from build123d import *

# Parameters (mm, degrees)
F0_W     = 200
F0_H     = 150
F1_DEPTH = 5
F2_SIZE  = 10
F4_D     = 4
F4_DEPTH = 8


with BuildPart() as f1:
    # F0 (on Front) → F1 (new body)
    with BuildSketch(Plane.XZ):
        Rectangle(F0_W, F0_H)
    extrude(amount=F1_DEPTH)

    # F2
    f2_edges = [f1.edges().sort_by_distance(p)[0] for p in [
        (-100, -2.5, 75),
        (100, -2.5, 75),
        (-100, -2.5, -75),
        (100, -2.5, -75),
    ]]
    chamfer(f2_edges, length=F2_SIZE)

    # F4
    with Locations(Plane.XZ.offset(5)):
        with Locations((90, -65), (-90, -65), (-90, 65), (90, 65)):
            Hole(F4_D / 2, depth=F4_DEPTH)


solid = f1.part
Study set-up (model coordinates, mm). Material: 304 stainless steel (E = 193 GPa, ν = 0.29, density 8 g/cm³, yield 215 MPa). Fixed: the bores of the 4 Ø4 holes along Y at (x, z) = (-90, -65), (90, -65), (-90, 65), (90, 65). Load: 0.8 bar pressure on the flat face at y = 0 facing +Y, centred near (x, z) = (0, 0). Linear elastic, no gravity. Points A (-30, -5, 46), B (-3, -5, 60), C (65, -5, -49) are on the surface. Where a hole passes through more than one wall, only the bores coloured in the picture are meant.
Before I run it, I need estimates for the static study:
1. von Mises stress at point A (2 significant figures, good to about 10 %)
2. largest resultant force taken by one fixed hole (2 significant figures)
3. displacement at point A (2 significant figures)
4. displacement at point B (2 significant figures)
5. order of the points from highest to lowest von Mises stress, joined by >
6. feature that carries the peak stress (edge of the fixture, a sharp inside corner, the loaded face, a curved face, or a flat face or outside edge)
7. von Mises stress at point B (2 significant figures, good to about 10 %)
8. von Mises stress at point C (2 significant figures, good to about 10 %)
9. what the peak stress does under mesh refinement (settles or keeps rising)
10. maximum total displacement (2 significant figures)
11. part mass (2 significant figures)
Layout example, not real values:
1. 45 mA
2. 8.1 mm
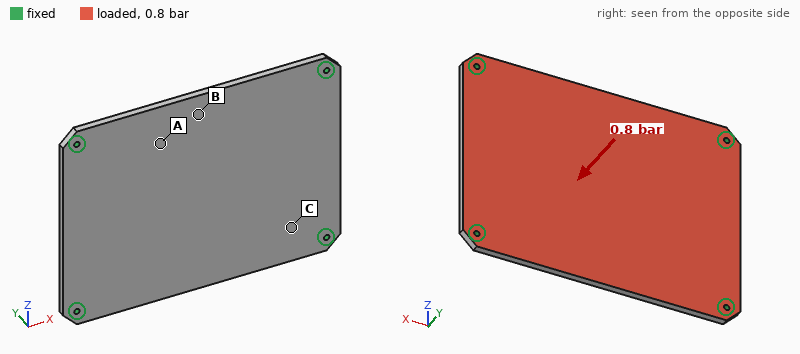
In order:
1. 26 MPa
2. 600 N
3. 0.17 mm
4. 0.19 mm
5. B > A > C
6. edge of the fixture
7. 36 MPa
8. 11 MPa
9. keeps rising
10. 0.22 mm
11. 1.2 kg
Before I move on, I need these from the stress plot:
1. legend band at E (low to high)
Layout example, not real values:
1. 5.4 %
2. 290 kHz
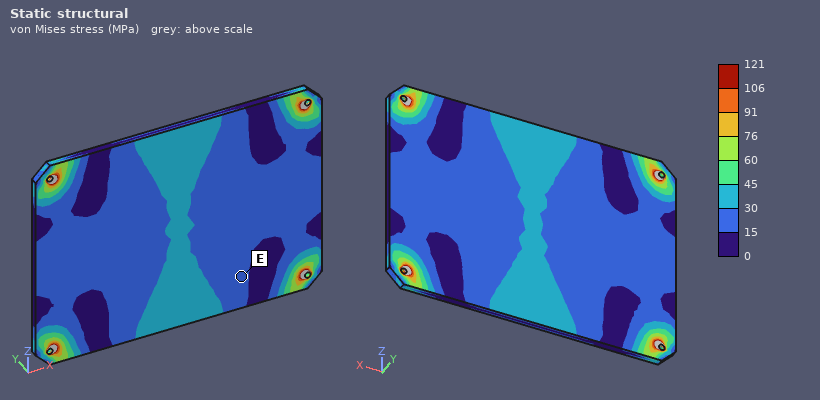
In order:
1. 15 to 30 MPa
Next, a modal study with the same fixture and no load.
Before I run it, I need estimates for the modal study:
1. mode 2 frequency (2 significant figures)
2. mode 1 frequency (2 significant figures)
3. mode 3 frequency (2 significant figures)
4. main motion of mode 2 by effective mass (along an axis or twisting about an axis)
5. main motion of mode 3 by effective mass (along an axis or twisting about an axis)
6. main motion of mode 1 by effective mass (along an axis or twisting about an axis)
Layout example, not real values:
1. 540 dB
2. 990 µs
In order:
1. 940 Hz
2. 560 Hz
3. 1300 Hz
4. twisting about X
5. twisting about Z
6. along Y
